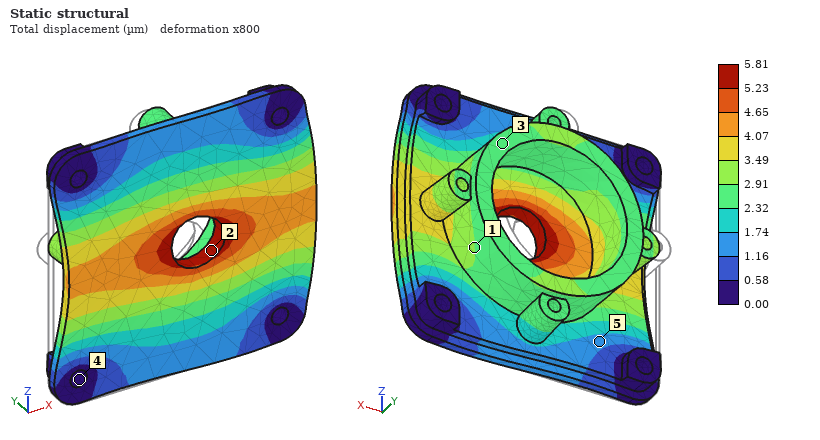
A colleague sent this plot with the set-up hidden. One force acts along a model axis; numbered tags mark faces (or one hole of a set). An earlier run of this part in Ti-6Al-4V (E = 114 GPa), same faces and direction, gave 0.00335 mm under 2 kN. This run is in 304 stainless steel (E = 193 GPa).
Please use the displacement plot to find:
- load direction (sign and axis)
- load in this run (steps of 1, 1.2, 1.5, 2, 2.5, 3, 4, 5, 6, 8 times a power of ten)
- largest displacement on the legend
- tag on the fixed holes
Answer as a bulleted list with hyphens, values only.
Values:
- +X
- 6 kN
- 5.81 µm
- 4
